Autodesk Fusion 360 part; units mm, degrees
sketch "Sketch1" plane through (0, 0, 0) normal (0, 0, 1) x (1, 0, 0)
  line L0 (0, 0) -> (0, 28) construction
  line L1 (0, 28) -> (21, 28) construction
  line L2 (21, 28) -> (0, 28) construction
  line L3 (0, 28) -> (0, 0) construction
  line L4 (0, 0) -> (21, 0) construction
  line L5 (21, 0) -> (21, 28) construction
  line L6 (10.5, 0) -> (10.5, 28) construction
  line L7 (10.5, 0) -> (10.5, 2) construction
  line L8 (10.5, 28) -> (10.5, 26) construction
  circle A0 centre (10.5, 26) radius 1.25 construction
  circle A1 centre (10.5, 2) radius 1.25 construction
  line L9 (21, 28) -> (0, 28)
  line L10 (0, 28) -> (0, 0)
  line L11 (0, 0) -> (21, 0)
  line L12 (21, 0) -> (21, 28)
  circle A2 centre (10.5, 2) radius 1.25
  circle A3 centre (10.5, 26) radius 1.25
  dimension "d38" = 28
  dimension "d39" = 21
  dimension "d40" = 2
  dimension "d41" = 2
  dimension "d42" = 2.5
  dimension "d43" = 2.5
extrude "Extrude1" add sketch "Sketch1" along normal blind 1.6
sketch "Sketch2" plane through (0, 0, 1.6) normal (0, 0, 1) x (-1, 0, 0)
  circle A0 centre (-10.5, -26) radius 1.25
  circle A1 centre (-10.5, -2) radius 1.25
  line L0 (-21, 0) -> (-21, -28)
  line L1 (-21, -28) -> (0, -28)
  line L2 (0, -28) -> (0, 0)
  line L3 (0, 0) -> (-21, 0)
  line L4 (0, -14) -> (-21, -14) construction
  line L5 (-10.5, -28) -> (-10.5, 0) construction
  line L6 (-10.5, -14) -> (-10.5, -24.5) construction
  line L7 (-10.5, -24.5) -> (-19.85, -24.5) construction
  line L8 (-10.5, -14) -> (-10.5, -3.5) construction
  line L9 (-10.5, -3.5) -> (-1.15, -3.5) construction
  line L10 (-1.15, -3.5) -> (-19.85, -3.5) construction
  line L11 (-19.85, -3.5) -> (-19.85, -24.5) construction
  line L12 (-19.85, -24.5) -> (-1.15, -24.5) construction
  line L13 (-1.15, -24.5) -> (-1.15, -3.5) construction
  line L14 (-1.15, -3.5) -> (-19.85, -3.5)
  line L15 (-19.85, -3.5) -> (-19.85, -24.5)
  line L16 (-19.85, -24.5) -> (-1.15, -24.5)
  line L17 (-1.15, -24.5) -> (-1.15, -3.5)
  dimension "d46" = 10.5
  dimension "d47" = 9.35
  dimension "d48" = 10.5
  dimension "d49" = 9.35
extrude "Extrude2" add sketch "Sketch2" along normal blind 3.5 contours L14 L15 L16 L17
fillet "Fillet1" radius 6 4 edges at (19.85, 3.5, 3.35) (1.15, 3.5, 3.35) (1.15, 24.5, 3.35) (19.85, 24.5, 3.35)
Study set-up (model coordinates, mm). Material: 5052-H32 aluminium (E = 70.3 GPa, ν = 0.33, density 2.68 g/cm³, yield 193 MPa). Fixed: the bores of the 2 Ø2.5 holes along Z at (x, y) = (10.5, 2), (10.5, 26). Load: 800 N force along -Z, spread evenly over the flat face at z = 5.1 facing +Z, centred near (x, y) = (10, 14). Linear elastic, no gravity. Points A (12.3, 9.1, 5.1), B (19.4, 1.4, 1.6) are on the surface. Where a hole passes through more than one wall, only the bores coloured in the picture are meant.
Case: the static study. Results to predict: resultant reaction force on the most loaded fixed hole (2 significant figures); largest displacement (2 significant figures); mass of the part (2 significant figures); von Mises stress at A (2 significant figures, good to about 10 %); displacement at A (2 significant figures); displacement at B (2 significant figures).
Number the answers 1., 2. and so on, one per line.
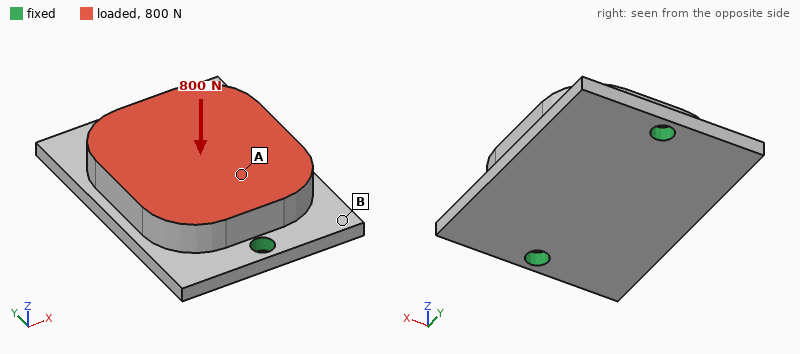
1. 520 N
2. 13 µm
3. 5.9 g
4. 25 MPa
5. 8.6 µm
6. 5.7 µm
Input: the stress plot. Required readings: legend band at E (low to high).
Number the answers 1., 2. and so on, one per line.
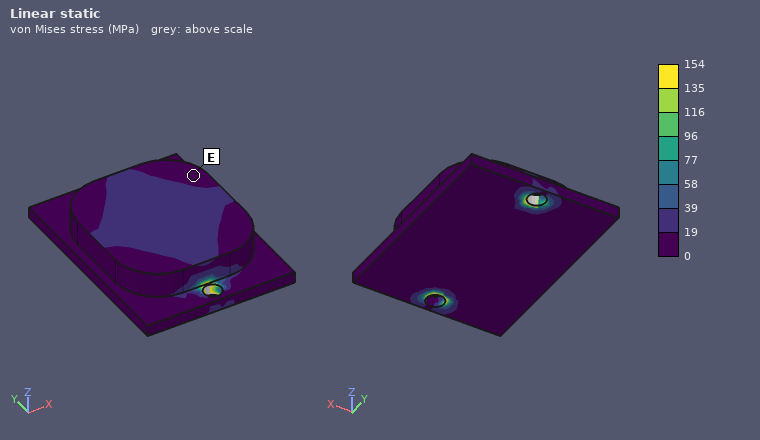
1. 0 to 19 MPa
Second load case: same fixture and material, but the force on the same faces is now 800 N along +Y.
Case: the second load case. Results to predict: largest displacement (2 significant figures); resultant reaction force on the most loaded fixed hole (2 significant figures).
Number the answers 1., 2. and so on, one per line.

1. 3.0 µm
2. 430 N
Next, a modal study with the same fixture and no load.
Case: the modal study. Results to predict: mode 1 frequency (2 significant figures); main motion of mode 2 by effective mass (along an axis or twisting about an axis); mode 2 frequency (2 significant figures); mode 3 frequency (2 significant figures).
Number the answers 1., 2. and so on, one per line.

1. 8300 Hz
2. along Z
3. 20 kHz
4. 31 kHz
